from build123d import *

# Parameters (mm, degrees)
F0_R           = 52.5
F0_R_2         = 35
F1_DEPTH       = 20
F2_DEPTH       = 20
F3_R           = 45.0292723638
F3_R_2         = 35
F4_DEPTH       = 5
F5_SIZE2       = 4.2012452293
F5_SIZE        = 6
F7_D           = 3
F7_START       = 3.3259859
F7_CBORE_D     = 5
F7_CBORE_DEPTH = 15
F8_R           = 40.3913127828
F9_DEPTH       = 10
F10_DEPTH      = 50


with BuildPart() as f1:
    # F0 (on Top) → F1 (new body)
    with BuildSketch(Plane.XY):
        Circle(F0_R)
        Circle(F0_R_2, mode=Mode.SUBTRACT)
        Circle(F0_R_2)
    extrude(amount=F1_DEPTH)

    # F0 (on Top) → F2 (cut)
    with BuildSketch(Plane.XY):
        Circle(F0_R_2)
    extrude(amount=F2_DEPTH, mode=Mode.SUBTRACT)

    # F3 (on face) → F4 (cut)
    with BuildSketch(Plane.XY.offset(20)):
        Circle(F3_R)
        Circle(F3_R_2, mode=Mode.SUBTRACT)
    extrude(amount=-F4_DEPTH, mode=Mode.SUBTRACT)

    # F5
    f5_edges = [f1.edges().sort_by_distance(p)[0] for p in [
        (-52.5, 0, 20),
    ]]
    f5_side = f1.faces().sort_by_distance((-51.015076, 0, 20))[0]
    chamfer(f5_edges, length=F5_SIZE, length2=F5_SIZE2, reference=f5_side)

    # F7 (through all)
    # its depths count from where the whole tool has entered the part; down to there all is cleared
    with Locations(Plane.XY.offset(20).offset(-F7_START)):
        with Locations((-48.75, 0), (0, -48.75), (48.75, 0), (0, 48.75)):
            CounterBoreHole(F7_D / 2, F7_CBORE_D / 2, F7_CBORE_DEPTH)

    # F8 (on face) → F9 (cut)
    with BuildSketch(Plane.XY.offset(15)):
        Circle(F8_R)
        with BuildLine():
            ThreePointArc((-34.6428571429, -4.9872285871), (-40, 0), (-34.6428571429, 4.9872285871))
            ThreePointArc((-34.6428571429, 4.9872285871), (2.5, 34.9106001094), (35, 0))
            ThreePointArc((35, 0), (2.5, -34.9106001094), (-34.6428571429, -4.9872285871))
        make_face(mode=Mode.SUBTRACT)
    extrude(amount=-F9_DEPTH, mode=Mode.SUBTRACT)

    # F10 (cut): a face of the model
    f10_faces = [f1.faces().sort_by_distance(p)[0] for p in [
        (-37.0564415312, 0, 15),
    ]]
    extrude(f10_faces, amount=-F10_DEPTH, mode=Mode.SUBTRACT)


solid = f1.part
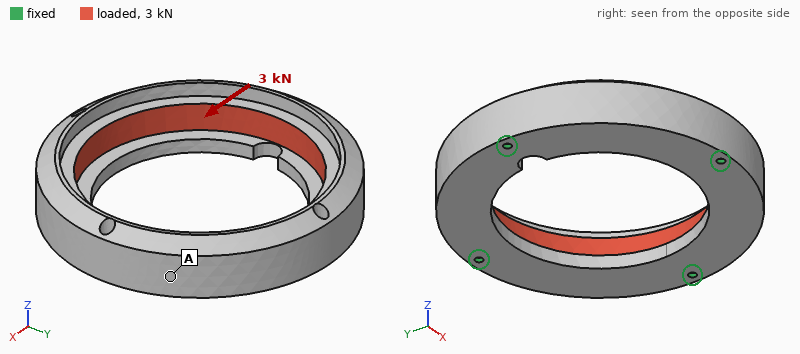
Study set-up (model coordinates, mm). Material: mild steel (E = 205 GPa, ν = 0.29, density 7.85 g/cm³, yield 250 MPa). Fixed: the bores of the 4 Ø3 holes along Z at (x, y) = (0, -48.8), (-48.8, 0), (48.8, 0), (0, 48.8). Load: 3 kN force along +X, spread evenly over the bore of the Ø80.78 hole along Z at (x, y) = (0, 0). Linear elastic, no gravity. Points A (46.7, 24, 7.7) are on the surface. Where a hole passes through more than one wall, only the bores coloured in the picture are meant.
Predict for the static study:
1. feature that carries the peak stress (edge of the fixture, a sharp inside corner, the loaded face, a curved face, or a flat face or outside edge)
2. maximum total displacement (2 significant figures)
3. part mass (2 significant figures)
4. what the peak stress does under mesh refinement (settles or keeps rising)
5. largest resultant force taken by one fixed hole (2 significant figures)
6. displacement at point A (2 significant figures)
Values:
edge of the fixture
3.4 µm
510 g
keeps rising
1.0 kN
2.3 µm
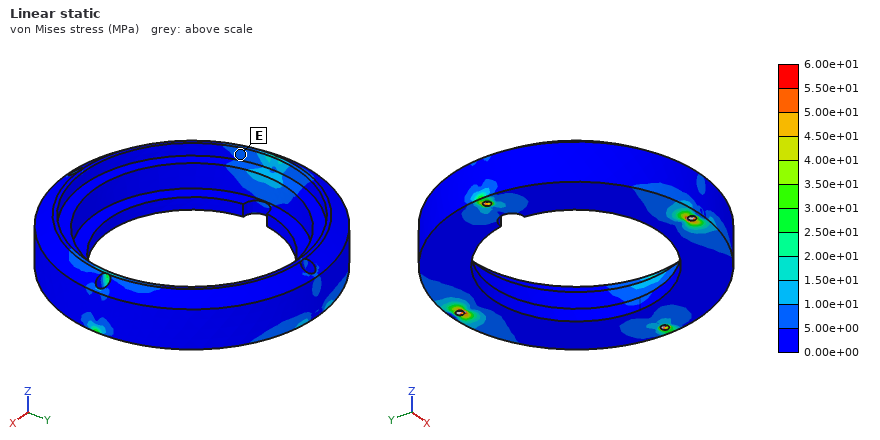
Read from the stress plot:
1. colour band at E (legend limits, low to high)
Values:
5.00e+00 to 1.00e+01 MPa
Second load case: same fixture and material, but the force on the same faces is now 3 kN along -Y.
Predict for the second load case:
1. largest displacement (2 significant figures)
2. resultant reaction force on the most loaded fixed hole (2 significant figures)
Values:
3.4 µm
1.0 kN
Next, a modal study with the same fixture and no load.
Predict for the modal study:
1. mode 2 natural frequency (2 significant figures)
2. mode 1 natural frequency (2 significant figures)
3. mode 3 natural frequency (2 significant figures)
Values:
6300 Hz
3800 Hz
6300 Hz
